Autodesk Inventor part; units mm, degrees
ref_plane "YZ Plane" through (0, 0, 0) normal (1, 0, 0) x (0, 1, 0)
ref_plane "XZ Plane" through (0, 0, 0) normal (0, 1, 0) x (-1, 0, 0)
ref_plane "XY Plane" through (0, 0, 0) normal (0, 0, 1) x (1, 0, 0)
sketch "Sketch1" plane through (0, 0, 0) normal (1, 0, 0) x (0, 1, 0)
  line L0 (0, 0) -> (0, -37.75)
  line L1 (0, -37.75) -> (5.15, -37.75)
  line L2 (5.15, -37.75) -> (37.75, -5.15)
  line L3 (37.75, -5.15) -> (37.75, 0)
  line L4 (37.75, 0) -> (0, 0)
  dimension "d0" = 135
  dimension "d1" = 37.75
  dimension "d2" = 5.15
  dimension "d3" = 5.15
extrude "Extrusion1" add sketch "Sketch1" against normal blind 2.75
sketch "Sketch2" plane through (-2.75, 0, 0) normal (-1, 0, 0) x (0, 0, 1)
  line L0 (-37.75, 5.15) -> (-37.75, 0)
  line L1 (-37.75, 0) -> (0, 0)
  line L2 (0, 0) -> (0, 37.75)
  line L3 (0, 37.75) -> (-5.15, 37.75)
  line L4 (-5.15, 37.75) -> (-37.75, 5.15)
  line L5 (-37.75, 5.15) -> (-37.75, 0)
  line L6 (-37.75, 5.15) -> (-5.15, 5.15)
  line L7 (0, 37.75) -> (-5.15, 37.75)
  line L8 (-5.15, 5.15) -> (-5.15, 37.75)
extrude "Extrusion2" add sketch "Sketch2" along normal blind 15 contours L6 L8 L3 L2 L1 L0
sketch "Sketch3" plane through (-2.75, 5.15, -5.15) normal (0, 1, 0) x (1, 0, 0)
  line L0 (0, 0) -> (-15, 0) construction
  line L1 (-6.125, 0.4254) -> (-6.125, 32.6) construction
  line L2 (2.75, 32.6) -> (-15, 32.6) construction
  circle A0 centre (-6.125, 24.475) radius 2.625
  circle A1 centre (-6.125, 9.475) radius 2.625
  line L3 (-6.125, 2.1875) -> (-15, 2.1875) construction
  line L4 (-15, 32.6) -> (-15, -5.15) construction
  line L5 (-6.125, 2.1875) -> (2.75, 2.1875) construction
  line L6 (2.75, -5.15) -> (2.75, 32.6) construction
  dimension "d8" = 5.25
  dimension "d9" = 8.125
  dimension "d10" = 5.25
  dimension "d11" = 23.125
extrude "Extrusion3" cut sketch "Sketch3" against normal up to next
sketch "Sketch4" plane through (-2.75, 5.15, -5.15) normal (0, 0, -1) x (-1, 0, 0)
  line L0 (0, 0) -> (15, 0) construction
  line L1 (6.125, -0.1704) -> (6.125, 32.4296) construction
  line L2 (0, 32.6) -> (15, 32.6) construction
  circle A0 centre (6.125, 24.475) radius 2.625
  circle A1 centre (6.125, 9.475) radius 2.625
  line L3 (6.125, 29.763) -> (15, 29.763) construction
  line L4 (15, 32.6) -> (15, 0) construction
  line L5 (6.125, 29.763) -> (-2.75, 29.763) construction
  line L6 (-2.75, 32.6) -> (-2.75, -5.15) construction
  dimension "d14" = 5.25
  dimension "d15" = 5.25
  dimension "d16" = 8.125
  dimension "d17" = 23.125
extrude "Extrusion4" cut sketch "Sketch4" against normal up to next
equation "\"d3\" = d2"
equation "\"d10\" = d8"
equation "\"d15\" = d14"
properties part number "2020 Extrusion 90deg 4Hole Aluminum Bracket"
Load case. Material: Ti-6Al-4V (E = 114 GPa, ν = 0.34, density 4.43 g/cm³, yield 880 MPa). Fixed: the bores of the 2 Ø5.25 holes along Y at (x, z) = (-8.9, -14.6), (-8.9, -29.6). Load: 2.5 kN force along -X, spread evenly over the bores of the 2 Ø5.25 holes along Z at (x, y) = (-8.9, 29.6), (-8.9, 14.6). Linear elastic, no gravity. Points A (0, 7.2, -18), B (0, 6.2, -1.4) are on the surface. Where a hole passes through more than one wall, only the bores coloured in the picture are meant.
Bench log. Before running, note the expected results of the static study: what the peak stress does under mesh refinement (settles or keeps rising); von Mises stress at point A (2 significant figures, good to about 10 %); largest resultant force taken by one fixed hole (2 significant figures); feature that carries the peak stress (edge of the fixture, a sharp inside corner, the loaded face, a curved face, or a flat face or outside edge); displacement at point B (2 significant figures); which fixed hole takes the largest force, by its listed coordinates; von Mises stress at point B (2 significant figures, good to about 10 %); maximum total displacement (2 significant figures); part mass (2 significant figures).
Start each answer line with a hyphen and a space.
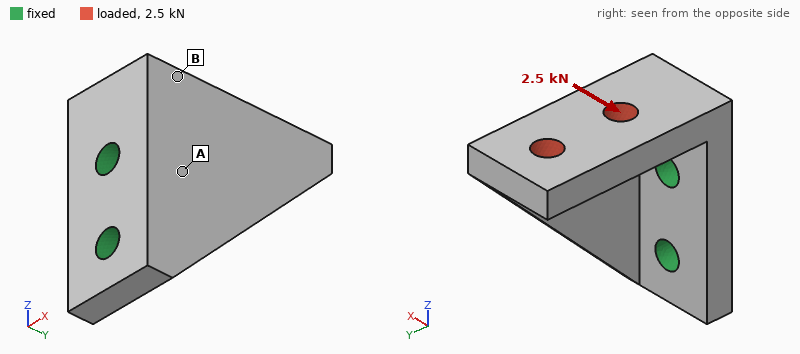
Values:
- keeps rising
- 180 MPa
- 3.5 kN
- edge of the fixture
- 0.096 mm
- (-8.9, -14.6)
- 81 MPa
- 0.42 mm
- 33 g
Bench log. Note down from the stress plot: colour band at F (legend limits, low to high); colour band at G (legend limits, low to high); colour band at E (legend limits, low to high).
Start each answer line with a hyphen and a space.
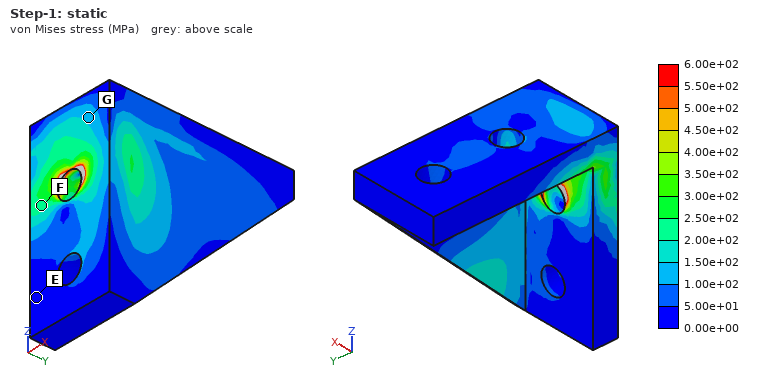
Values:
- 2.00e+02 to 2.50e+02 MPa
- 1.00e+02 to 1.50e+02 MPa
- 0.00e+00 to 5.00e+01 MPa
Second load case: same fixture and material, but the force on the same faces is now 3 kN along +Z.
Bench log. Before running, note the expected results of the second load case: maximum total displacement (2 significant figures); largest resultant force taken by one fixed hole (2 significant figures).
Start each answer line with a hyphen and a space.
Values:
- 0.34 mm
- 3.0 kN
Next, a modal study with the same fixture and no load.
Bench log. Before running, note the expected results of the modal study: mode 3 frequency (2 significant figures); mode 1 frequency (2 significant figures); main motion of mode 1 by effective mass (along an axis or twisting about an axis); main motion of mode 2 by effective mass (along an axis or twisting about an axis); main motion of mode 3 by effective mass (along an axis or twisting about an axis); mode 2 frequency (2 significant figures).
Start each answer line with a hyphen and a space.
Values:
- 11 kHz
- 3800 Hz
- along X
- along Z
- along Y
- 5700 Hz
